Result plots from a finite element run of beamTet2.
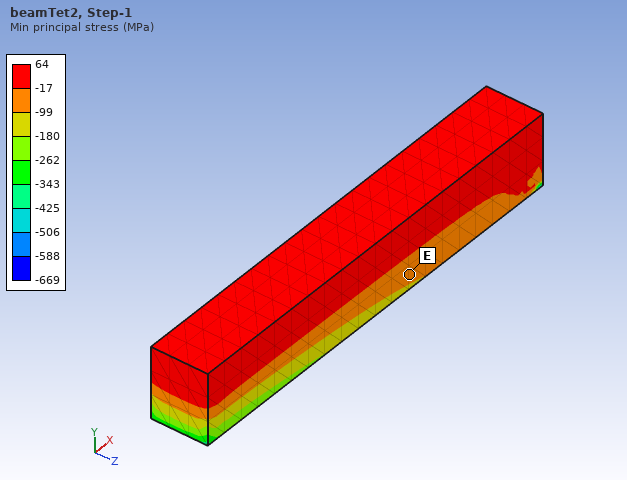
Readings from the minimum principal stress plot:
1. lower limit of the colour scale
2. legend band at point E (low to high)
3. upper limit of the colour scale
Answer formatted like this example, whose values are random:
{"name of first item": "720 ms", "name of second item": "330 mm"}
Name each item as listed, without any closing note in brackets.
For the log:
{"lower limit of the colour scale": "-669 MPa", "legend band at point E": "-99 to -17 MPa", "upper limit of the colour scale": "64 MPa"}
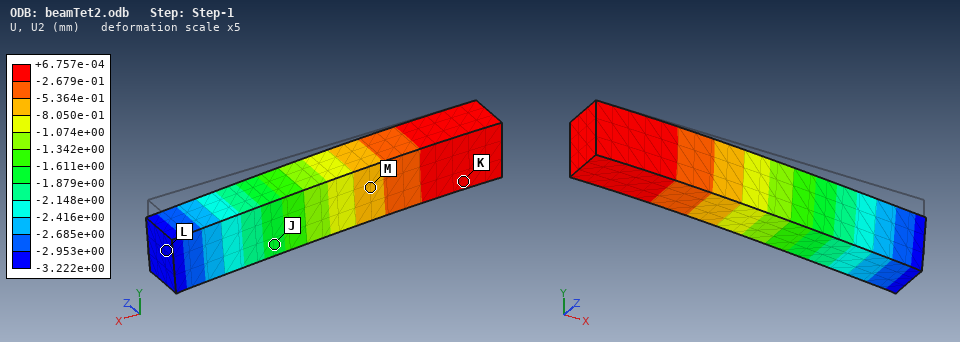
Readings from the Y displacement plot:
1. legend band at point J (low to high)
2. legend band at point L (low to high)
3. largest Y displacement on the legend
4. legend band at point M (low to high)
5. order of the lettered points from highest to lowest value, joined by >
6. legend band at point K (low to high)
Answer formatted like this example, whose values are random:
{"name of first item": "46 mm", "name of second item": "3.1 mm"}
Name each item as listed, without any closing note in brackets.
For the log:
{"legend band at point J": "-1.879e+00 to -1.611e+00 mm", "legend band at point L": "-3.222e+00 to -2.953e+00 mm", "largest Y displacement on the legend": "+6.757e-04 mm", "legend band at point M": "-8.050e-01 to -5.364e-01 mm", "order of the lettered points from highest to lowest value, joined by >": "K > M > J > L", "legend band at point K": "-2.679e-01 to +6.757e-04 mm"}
